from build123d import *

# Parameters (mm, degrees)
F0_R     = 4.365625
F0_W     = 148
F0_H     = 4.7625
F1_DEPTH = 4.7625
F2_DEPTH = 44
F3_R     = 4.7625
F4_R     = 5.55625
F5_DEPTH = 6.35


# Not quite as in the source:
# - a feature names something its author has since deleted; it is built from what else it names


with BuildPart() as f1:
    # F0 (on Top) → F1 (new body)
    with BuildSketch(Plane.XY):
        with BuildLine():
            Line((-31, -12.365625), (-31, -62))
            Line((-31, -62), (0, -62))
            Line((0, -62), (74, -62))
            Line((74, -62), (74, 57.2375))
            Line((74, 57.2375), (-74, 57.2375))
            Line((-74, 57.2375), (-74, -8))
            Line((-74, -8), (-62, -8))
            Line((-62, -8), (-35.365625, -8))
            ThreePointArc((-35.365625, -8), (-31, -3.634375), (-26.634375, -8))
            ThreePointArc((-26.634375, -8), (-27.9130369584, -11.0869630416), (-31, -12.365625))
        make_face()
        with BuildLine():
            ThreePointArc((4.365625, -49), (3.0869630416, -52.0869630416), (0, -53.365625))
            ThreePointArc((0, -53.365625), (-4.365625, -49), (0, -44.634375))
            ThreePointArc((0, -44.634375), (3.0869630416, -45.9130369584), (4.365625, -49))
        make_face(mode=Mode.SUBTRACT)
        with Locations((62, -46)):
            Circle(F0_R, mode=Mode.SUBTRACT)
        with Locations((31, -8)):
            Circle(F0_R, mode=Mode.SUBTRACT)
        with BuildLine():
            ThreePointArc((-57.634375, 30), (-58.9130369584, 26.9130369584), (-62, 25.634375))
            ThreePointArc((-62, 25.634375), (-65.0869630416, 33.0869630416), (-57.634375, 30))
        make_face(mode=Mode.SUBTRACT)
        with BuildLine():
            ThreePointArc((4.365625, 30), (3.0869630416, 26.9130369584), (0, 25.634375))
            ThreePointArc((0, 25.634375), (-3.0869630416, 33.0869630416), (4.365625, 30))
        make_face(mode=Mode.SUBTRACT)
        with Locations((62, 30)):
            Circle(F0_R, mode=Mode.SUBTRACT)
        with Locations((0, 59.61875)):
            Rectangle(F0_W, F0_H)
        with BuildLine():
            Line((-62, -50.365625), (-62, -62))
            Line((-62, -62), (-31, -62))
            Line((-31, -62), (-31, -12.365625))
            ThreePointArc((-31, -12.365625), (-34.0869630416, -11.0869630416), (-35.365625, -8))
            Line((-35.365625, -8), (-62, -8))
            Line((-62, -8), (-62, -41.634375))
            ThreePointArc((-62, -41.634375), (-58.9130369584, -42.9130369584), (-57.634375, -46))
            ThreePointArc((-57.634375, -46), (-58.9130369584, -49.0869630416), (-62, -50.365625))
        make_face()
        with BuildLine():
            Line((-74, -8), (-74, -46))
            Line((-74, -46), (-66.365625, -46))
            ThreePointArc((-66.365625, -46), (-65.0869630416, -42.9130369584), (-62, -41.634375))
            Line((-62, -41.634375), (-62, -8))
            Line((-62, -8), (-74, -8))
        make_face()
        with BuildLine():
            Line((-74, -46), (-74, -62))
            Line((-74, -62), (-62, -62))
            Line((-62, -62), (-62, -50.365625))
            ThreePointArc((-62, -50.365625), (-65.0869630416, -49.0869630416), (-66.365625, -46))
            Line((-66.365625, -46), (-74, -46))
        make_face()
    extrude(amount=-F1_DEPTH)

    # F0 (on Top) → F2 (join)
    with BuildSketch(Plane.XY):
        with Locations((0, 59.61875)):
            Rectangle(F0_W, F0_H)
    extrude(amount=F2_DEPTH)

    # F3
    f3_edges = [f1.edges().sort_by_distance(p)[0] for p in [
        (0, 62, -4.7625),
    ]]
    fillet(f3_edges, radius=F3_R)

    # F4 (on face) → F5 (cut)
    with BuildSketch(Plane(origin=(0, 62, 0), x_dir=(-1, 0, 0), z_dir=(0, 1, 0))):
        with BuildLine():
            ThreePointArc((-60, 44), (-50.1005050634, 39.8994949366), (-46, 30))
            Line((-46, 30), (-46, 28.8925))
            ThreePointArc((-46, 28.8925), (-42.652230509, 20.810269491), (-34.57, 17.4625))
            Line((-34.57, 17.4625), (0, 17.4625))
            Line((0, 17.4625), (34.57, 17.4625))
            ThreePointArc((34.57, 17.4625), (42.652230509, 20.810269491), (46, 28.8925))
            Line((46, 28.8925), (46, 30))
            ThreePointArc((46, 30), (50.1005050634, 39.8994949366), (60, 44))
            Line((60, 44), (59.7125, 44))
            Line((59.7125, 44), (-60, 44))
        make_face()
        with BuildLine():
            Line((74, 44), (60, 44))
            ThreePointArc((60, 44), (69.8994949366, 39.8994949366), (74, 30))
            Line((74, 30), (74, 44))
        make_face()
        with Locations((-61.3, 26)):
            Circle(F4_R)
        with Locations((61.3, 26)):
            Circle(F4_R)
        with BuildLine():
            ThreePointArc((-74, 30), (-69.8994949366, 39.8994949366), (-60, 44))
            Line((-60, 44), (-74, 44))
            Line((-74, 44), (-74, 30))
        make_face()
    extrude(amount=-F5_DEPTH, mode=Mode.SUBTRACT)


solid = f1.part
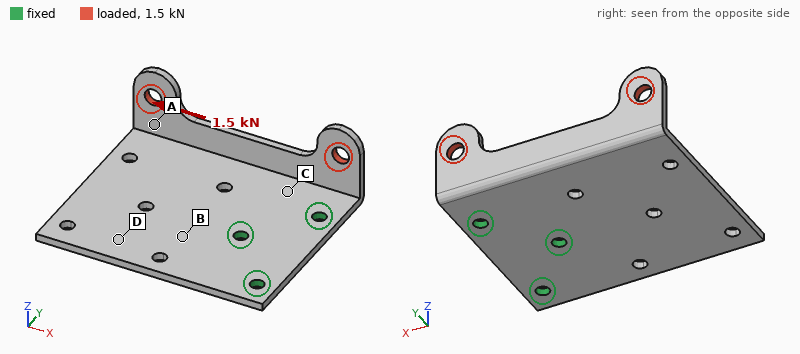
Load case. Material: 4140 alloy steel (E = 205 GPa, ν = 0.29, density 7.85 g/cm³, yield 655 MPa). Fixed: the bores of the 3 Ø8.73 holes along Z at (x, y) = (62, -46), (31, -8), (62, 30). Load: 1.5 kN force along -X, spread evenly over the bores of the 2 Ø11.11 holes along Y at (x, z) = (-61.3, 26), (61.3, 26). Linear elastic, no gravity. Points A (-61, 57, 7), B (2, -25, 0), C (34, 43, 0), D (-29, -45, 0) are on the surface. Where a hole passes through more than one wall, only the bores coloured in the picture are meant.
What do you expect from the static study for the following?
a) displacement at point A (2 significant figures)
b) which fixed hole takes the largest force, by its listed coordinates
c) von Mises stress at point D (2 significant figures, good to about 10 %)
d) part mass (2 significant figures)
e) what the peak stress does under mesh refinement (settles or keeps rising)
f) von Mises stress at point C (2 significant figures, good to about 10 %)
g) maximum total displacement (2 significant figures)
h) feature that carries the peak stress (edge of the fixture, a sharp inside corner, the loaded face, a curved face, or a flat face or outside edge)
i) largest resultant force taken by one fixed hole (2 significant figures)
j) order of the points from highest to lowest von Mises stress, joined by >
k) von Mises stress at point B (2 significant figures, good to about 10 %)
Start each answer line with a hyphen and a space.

- 0.51 mm
- (62, 30)
- 21 MPa
- 800 g
- keeps rising
- 50 MPa
- 0.63 mm
- edge of the fixture
- 1.7 kN
- C > B > D > A
- 37 MPa
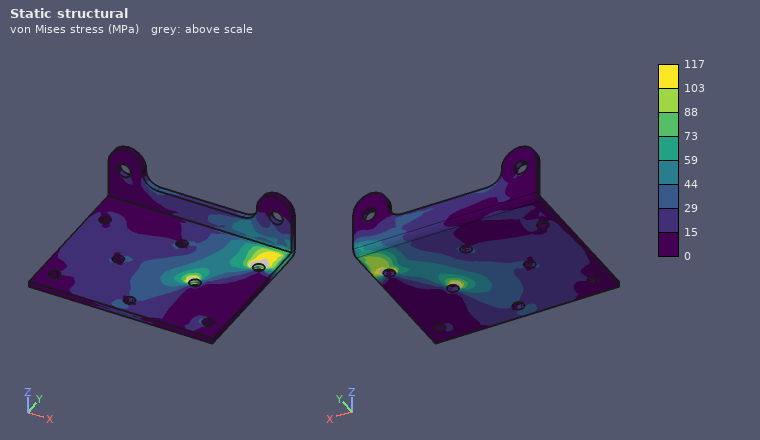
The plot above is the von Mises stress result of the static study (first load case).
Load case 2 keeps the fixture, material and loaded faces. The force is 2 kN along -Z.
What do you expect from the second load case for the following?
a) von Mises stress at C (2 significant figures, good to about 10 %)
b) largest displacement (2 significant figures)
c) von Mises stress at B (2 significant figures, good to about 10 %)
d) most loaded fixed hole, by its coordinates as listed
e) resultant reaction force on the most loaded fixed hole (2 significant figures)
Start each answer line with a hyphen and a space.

- 110 MPa
- 1.9 mm
- 120 MPa
- (62, 30)
- 1.5 kN
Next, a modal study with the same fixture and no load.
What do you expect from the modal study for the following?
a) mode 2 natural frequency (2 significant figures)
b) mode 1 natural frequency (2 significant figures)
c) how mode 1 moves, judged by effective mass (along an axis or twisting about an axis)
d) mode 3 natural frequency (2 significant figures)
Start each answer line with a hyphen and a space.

- 520 Hz
- 330 Hz
- along Z
- 1300 Hz
